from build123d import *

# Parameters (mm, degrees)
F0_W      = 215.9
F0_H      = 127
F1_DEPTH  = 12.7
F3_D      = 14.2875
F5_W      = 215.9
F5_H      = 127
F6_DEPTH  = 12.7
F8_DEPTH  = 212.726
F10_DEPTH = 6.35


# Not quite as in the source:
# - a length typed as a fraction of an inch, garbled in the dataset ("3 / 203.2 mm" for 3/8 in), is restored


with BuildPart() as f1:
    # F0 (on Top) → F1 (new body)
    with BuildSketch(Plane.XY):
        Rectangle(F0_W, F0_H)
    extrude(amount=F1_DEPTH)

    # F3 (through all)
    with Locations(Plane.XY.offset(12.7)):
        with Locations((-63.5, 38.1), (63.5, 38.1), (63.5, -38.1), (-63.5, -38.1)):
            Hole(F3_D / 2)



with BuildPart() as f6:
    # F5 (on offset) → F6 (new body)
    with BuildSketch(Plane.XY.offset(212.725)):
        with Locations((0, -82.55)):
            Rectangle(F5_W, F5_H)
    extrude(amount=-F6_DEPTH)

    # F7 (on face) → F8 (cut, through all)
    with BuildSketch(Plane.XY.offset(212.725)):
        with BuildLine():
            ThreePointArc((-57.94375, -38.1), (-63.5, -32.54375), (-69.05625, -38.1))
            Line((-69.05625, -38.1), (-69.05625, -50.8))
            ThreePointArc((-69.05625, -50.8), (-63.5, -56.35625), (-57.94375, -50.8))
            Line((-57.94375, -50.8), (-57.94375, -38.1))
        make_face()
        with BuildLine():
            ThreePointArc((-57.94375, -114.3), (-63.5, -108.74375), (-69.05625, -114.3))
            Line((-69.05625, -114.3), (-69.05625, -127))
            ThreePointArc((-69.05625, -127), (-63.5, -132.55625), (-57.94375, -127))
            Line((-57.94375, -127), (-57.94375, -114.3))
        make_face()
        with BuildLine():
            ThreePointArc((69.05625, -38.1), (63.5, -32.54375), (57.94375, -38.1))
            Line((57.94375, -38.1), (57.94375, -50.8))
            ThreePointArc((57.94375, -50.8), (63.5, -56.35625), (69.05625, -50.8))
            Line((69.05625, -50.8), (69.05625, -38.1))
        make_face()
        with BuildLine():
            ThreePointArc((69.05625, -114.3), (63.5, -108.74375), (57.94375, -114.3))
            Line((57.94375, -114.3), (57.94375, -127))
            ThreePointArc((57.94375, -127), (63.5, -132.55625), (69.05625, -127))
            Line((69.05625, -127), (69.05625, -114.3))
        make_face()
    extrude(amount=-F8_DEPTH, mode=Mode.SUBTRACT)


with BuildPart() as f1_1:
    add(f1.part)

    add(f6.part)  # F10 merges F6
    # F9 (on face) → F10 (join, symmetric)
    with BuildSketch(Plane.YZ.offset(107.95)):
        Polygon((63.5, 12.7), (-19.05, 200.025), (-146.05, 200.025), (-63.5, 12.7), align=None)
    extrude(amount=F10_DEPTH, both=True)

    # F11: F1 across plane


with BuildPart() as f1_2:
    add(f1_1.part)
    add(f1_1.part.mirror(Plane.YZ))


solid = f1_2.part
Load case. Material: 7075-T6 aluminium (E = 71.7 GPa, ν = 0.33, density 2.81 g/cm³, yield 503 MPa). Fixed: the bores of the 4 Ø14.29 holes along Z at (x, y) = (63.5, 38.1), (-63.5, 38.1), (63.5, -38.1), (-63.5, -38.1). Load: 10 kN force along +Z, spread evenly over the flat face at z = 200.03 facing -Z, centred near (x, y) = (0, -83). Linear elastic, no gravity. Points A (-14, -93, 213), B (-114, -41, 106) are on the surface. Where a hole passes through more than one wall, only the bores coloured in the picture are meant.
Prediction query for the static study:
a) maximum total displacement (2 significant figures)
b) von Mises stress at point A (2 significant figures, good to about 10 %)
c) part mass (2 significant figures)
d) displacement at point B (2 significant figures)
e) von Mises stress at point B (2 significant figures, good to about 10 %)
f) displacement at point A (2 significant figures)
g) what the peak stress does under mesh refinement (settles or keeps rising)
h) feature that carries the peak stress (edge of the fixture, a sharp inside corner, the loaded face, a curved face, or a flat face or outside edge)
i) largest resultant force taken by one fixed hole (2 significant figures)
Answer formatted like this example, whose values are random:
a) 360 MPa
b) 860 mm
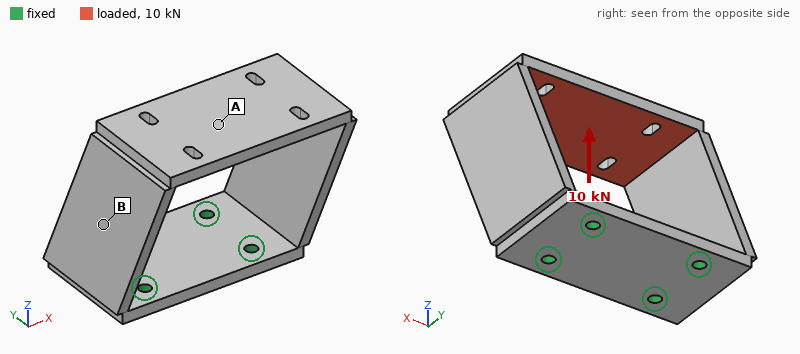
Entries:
a) 1.2 mm
b) 49 MPa
c) 3.6 kg
d) 0.38 mm
e) 14 MPa
f) 1.0 mm
g) keeps rising
h) edge of the fixture
i) 7.3 kN
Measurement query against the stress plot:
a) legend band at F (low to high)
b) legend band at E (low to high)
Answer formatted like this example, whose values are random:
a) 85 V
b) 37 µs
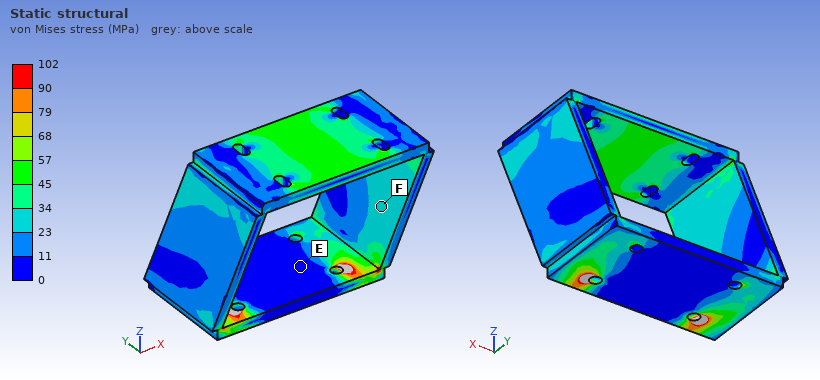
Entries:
a) 23 to 34 MPa
b) 0 to 11 MPa
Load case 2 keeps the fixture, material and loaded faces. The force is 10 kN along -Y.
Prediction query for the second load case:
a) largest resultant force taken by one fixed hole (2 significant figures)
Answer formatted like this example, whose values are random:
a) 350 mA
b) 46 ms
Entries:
a) 12 kN
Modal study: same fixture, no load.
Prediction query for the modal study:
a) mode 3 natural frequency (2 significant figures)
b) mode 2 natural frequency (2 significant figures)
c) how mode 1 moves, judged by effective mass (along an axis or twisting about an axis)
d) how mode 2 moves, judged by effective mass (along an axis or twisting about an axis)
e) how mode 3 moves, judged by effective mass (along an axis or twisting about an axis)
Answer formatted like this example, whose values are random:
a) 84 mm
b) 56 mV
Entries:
a) 510 Hz
b) 330 Hz
c) along X
d) along Y
e) twisting about Z
